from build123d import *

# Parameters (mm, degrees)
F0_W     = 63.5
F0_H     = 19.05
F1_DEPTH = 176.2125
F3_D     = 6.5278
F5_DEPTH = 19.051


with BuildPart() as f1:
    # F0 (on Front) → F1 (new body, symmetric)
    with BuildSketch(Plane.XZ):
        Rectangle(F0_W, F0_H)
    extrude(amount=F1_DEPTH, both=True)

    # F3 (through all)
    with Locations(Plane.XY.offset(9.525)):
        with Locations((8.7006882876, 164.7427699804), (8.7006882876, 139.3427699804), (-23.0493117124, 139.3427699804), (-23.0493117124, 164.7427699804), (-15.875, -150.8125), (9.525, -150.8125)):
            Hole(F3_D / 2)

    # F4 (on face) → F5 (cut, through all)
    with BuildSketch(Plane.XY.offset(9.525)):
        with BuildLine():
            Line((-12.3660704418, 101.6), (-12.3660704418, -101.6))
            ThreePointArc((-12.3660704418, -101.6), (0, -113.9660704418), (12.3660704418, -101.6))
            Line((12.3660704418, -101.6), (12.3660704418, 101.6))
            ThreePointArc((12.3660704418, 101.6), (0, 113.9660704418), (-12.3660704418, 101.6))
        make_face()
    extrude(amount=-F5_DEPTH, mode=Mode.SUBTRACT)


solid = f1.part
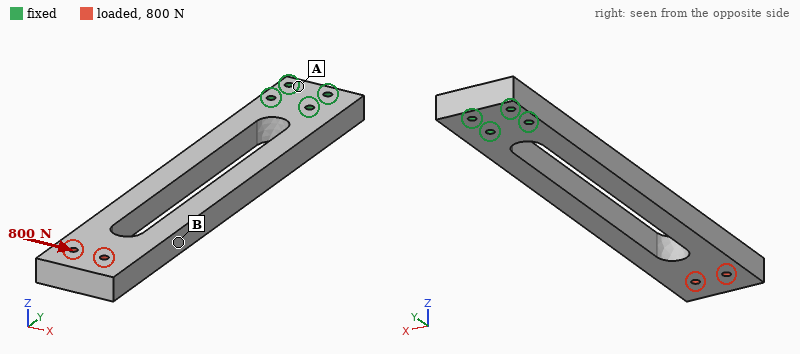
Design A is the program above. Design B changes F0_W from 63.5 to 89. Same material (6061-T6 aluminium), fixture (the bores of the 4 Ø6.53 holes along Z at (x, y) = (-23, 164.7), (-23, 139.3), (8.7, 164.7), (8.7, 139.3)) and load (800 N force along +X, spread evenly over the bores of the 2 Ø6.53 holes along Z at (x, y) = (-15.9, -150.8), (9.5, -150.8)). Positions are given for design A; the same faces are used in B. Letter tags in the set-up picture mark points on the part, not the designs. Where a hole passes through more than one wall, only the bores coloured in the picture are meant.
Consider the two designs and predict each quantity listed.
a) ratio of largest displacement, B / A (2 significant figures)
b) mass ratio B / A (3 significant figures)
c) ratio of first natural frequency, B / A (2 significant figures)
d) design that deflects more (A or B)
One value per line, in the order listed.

0.32
1.54
1.0
A
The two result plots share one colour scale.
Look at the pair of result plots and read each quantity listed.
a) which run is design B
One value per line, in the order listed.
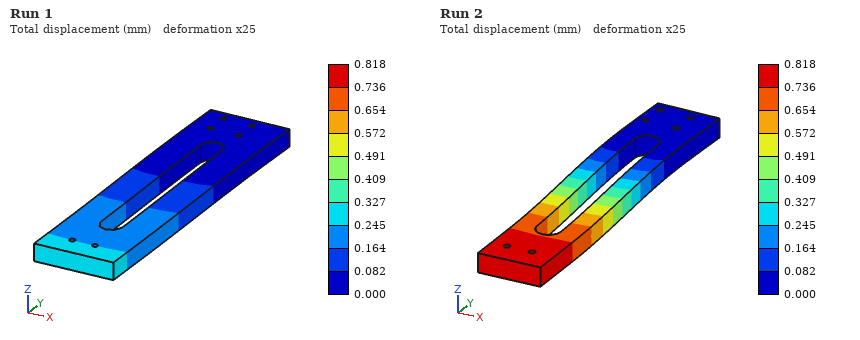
Run 1
